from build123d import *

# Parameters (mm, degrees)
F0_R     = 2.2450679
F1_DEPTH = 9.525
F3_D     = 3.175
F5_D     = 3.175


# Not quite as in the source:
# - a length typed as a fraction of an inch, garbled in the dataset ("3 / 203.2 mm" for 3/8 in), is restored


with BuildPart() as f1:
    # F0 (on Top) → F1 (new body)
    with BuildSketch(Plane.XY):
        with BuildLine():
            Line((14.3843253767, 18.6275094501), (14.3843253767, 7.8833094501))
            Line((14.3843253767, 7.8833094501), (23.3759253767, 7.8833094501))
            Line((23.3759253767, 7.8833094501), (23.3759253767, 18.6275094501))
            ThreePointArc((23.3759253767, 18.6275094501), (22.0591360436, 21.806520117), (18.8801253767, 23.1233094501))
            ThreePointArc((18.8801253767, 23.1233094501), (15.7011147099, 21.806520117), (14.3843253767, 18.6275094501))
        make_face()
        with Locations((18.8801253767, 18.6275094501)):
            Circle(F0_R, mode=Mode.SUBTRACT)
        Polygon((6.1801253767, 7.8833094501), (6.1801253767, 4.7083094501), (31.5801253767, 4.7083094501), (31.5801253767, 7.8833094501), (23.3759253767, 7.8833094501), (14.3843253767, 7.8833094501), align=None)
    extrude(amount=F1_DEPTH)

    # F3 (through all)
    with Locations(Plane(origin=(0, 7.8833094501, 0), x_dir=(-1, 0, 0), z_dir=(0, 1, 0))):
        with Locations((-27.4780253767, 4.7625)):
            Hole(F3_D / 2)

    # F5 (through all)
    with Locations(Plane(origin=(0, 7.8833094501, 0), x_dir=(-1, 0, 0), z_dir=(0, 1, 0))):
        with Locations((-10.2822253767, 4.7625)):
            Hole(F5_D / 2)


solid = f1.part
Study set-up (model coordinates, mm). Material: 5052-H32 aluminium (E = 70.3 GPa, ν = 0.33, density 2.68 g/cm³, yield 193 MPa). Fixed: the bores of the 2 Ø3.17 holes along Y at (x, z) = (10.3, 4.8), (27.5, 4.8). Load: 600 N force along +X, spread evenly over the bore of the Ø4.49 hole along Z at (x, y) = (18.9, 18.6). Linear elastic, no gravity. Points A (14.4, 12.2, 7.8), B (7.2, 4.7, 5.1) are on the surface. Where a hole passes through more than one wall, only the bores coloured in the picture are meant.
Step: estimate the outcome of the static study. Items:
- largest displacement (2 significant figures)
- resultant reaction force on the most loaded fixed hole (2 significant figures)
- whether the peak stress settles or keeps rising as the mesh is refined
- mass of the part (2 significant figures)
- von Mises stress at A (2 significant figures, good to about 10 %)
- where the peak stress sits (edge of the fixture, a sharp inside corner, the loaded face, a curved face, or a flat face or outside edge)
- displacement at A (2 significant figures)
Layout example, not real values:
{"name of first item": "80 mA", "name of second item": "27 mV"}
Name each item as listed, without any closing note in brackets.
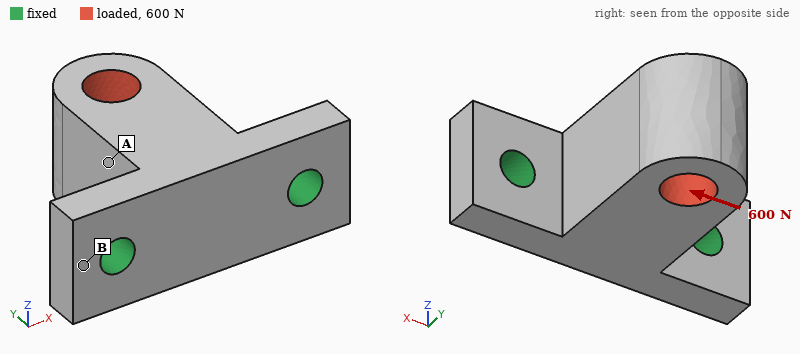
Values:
{"largest displacement": "36 µm", "resultant reaction force on the most loaded fixed hole": "660 N", "whether the peak stress settles or keeps rising as the mesh is refined": "keeps rising", "mass of the part": "4.8 g", "von Mises stress at A": "31 MPa", "where the peak stress sits": "edge of the fixture", "displacement at A": "12 µm"}
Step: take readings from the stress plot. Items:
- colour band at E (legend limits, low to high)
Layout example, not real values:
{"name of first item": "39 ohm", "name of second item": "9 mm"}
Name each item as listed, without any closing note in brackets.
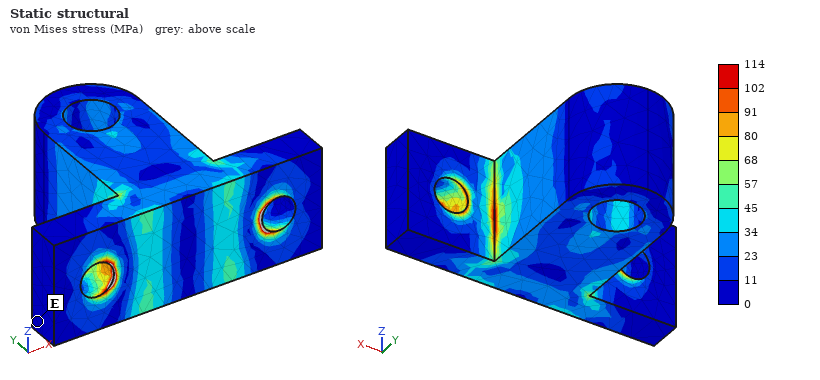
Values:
{"colour band at E": "0 to 11 MPa"}
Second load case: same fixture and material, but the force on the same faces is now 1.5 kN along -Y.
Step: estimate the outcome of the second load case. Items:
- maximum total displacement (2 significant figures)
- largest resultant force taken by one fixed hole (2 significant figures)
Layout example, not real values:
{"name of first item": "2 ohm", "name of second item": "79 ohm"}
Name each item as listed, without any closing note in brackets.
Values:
{"maximum total displacement": "15 µm", "largest resultant force taken by one fixed hole": "790 N"}
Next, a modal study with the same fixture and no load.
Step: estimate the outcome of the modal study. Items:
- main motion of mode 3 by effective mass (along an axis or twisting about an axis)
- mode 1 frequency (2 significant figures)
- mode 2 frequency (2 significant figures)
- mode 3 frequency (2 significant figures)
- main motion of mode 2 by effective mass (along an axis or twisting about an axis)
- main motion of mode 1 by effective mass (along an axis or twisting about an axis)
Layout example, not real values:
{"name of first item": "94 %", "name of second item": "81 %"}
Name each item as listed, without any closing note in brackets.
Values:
{"main motion of mode 3 by effective mass": "along Y", "mode 1 frequency": "10 kHz", "mode 2 frequency": "19 kHz", "mode 3 frequency": "31 kHz", "main motion of mode 2 by effective mass": "along X", "main motion of mode 1 by effective mass": "along Z"}
